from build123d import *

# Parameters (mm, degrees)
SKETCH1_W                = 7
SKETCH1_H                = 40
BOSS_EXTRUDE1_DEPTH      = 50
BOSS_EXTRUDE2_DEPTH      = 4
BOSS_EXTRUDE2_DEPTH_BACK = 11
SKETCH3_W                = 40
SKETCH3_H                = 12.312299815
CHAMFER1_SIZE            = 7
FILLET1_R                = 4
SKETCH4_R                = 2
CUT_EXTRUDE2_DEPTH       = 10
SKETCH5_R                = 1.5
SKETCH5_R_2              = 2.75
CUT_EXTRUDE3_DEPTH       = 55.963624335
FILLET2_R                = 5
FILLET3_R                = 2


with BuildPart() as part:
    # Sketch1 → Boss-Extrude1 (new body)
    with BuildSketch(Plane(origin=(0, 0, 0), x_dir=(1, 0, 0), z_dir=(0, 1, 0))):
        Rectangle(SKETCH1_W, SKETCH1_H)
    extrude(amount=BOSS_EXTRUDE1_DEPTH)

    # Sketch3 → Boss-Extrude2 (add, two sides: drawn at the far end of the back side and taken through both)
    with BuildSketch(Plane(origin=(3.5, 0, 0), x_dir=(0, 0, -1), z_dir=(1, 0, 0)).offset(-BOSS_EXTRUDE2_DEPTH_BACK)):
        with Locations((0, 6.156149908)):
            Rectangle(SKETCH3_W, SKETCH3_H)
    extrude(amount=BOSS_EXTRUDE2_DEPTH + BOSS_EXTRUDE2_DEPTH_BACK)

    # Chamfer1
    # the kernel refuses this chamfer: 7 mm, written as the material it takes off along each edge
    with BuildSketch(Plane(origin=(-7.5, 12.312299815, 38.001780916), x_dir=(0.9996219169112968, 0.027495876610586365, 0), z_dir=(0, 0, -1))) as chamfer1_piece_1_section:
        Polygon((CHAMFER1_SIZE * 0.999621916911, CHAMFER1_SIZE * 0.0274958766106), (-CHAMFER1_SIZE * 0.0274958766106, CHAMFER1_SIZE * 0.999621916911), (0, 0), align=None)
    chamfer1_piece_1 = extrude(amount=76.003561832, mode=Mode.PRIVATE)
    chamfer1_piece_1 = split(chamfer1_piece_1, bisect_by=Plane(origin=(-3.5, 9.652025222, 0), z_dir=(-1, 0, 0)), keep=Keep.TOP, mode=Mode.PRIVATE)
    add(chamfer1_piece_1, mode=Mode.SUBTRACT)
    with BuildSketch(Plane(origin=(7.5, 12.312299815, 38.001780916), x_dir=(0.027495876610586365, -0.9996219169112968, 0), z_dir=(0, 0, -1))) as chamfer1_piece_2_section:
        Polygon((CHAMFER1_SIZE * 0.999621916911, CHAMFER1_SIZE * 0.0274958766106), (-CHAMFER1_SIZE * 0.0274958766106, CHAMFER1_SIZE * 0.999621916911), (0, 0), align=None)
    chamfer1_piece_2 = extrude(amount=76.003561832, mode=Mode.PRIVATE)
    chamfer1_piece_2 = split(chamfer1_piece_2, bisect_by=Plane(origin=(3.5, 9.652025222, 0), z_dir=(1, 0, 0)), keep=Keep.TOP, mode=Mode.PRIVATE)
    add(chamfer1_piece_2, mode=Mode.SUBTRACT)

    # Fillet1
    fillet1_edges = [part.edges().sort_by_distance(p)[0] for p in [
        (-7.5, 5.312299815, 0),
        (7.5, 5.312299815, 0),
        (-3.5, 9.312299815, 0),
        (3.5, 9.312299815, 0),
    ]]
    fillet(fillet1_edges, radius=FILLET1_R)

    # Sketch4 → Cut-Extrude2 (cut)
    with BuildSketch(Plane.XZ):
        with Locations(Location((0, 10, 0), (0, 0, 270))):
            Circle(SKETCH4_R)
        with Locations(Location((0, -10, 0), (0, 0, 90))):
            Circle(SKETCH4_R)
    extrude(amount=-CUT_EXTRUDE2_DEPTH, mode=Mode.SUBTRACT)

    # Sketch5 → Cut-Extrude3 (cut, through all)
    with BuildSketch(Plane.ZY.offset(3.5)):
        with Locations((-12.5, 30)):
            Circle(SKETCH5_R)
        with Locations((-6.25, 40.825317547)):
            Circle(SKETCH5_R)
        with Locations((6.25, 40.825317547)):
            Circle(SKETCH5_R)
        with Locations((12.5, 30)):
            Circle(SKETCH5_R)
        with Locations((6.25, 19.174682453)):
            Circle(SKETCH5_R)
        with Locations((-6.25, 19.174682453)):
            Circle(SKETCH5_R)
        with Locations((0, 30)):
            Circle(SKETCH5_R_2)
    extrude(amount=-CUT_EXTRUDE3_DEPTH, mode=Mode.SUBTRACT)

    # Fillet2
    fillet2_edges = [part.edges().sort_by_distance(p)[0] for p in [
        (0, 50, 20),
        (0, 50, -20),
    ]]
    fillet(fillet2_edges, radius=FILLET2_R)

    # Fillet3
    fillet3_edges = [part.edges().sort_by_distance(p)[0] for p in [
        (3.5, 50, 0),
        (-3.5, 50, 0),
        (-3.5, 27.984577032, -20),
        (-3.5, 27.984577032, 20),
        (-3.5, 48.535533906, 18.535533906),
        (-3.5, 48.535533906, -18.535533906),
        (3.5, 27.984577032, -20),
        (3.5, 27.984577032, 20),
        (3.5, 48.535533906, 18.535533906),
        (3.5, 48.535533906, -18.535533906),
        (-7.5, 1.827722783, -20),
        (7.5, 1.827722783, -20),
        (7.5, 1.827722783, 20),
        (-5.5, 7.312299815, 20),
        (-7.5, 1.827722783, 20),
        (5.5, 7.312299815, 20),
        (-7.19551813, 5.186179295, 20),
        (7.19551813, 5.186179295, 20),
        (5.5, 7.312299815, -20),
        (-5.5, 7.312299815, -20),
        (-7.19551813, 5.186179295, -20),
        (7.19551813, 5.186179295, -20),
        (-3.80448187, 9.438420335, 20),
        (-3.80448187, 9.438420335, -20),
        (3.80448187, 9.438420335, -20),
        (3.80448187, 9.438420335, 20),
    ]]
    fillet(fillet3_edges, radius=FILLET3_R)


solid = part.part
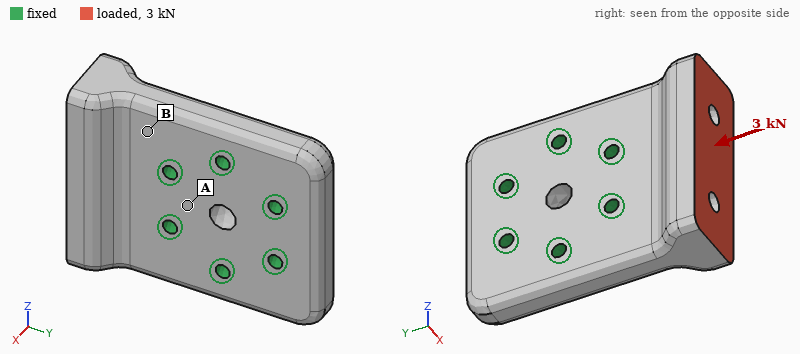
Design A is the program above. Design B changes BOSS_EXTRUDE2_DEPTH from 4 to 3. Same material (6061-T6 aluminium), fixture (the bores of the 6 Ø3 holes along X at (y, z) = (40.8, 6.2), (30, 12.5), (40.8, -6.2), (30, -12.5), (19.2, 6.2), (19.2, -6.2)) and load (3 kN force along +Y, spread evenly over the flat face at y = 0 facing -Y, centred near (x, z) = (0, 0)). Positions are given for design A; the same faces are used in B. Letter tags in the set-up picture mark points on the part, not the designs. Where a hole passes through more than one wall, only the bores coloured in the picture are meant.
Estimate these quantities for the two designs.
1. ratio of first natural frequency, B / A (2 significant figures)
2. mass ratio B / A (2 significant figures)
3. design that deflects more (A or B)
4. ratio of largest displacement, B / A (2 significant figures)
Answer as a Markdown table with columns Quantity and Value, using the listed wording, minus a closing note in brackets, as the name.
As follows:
| Quantity | Value |
|---|---|
| ratio of first natural frequency, B / A | 1.0 |
| mass ratio B / A | 0.98 |
| design that deflects more | B |
| ratio of largest displacement, B / A | 1.8 |
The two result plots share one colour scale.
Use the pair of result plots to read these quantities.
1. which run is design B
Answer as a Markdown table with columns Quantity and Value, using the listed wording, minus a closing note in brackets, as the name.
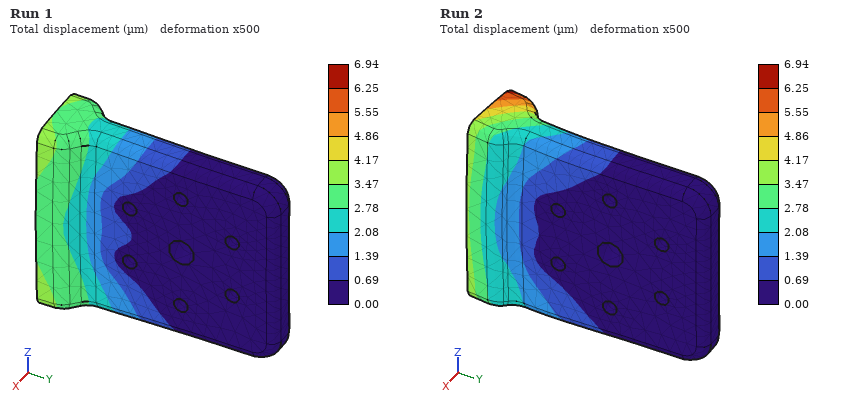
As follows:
| Quantity | Value |
|---|---|
| which run is design B | Run 2 |
